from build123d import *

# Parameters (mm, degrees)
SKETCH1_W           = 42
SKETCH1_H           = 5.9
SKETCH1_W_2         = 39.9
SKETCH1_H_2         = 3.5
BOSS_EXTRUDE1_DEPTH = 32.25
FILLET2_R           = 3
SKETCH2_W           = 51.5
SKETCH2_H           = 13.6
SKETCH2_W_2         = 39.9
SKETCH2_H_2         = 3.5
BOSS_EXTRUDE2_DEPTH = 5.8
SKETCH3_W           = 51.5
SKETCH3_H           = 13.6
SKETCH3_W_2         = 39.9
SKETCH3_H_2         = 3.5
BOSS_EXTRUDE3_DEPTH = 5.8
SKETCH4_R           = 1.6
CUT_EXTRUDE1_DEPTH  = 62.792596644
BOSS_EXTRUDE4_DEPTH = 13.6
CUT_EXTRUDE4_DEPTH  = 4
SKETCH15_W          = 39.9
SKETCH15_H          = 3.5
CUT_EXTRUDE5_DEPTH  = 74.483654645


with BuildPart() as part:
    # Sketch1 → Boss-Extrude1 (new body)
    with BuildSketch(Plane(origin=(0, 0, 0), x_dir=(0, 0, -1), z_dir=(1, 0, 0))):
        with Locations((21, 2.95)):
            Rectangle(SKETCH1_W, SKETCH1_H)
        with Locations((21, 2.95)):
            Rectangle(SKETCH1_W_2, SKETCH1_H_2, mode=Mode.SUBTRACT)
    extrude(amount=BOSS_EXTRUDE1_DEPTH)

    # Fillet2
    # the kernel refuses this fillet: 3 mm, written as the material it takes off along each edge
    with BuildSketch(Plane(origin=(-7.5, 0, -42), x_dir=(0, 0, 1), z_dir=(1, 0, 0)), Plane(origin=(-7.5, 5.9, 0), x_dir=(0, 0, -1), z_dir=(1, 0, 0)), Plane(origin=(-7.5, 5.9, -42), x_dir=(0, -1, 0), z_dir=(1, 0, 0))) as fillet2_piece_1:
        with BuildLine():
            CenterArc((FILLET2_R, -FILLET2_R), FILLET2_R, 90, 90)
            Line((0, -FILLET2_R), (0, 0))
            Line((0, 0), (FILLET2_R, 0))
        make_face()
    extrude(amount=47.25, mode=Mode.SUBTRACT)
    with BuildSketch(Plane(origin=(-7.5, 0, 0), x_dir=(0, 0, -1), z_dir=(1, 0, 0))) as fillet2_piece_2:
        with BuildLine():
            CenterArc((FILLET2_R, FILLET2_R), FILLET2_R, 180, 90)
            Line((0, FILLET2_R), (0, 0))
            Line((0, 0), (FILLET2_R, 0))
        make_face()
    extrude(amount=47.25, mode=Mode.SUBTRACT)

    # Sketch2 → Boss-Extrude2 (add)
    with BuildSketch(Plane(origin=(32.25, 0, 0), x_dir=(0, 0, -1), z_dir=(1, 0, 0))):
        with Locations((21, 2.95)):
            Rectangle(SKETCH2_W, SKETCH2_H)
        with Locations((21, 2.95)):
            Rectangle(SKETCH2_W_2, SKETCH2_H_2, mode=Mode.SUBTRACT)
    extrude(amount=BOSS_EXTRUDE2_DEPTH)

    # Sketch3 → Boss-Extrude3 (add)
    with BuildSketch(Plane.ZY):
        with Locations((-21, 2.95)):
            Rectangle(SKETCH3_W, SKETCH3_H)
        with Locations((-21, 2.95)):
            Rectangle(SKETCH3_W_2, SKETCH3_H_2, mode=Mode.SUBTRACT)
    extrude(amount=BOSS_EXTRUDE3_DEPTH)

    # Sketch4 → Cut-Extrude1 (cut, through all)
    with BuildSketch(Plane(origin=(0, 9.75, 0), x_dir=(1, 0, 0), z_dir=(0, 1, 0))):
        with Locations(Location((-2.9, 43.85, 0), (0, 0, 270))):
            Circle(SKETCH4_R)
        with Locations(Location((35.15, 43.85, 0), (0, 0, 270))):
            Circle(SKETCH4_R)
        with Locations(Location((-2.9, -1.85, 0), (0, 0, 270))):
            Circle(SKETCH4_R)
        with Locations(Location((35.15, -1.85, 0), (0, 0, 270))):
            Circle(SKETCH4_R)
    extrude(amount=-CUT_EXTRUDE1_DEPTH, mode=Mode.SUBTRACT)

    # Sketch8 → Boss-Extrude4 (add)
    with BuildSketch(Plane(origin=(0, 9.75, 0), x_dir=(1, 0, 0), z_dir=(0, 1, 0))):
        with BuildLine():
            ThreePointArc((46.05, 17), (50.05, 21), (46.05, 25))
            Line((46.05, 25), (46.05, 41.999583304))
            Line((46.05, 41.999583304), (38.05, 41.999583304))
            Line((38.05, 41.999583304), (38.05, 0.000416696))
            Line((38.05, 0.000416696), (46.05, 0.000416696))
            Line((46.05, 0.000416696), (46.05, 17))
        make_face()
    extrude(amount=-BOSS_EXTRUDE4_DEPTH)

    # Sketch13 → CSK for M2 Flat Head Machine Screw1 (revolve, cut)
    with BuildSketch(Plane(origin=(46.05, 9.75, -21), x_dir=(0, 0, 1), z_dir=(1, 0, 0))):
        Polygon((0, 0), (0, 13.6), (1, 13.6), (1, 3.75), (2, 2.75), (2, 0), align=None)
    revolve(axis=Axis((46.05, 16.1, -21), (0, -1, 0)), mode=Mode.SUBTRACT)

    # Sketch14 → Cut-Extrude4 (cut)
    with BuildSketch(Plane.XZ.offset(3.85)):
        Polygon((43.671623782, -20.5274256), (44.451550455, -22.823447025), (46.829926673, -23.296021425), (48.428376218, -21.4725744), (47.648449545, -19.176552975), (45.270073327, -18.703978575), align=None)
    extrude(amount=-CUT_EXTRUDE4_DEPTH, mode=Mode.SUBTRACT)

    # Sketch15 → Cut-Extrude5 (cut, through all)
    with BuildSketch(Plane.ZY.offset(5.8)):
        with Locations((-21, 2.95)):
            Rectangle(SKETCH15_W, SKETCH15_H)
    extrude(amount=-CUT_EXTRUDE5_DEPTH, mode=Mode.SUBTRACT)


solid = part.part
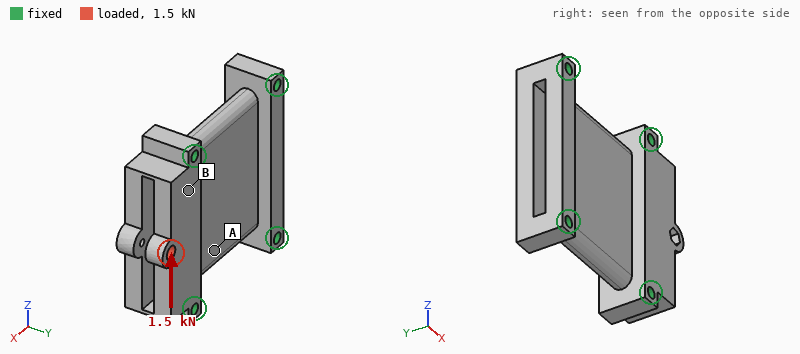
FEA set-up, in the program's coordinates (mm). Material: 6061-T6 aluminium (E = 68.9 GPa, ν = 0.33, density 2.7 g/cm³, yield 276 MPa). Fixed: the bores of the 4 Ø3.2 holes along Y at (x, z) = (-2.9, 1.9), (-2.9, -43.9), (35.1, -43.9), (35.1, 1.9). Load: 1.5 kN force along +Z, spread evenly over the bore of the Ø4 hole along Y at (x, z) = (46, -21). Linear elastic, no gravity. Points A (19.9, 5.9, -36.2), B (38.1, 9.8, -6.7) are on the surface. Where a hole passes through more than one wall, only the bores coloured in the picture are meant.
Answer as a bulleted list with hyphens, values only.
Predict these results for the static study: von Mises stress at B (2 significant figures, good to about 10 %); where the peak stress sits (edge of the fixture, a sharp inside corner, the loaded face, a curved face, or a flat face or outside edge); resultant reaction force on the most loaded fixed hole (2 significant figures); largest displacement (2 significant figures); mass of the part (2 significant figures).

- 17 MPa
- a flat face or outside edge
- 830 N
- 19 µm
- 35 g
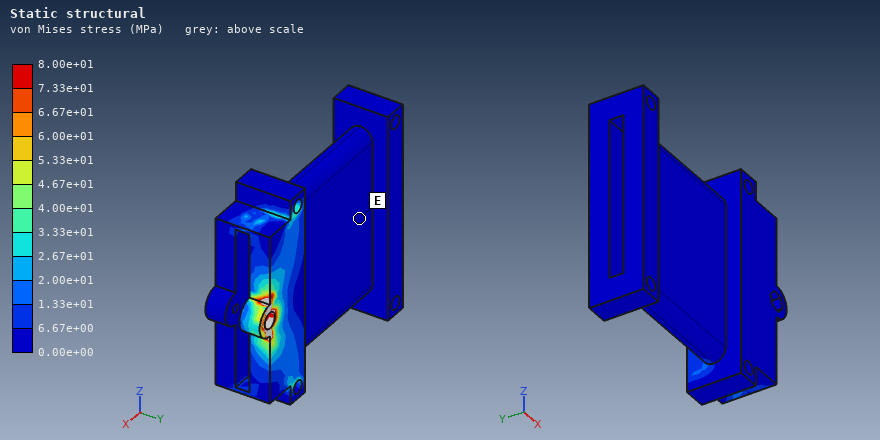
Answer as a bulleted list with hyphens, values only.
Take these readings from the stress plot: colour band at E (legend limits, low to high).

- 0.00e+00 to 6.67e+00 MPa
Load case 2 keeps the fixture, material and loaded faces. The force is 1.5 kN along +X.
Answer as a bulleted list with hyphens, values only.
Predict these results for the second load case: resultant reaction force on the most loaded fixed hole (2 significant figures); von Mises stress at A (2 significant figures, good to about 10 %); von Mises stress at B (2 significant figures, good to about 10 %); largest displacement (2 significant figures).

- 700 N
- 12 MPa
- 39 MPa
- 45 µm
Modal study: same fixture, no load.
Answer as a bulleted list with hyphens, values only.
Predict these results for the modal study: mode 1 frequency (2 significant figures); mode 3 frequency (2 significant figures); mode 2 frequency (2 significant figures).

- 6400 Hz
- 10 kHz
- 6500 Hz
